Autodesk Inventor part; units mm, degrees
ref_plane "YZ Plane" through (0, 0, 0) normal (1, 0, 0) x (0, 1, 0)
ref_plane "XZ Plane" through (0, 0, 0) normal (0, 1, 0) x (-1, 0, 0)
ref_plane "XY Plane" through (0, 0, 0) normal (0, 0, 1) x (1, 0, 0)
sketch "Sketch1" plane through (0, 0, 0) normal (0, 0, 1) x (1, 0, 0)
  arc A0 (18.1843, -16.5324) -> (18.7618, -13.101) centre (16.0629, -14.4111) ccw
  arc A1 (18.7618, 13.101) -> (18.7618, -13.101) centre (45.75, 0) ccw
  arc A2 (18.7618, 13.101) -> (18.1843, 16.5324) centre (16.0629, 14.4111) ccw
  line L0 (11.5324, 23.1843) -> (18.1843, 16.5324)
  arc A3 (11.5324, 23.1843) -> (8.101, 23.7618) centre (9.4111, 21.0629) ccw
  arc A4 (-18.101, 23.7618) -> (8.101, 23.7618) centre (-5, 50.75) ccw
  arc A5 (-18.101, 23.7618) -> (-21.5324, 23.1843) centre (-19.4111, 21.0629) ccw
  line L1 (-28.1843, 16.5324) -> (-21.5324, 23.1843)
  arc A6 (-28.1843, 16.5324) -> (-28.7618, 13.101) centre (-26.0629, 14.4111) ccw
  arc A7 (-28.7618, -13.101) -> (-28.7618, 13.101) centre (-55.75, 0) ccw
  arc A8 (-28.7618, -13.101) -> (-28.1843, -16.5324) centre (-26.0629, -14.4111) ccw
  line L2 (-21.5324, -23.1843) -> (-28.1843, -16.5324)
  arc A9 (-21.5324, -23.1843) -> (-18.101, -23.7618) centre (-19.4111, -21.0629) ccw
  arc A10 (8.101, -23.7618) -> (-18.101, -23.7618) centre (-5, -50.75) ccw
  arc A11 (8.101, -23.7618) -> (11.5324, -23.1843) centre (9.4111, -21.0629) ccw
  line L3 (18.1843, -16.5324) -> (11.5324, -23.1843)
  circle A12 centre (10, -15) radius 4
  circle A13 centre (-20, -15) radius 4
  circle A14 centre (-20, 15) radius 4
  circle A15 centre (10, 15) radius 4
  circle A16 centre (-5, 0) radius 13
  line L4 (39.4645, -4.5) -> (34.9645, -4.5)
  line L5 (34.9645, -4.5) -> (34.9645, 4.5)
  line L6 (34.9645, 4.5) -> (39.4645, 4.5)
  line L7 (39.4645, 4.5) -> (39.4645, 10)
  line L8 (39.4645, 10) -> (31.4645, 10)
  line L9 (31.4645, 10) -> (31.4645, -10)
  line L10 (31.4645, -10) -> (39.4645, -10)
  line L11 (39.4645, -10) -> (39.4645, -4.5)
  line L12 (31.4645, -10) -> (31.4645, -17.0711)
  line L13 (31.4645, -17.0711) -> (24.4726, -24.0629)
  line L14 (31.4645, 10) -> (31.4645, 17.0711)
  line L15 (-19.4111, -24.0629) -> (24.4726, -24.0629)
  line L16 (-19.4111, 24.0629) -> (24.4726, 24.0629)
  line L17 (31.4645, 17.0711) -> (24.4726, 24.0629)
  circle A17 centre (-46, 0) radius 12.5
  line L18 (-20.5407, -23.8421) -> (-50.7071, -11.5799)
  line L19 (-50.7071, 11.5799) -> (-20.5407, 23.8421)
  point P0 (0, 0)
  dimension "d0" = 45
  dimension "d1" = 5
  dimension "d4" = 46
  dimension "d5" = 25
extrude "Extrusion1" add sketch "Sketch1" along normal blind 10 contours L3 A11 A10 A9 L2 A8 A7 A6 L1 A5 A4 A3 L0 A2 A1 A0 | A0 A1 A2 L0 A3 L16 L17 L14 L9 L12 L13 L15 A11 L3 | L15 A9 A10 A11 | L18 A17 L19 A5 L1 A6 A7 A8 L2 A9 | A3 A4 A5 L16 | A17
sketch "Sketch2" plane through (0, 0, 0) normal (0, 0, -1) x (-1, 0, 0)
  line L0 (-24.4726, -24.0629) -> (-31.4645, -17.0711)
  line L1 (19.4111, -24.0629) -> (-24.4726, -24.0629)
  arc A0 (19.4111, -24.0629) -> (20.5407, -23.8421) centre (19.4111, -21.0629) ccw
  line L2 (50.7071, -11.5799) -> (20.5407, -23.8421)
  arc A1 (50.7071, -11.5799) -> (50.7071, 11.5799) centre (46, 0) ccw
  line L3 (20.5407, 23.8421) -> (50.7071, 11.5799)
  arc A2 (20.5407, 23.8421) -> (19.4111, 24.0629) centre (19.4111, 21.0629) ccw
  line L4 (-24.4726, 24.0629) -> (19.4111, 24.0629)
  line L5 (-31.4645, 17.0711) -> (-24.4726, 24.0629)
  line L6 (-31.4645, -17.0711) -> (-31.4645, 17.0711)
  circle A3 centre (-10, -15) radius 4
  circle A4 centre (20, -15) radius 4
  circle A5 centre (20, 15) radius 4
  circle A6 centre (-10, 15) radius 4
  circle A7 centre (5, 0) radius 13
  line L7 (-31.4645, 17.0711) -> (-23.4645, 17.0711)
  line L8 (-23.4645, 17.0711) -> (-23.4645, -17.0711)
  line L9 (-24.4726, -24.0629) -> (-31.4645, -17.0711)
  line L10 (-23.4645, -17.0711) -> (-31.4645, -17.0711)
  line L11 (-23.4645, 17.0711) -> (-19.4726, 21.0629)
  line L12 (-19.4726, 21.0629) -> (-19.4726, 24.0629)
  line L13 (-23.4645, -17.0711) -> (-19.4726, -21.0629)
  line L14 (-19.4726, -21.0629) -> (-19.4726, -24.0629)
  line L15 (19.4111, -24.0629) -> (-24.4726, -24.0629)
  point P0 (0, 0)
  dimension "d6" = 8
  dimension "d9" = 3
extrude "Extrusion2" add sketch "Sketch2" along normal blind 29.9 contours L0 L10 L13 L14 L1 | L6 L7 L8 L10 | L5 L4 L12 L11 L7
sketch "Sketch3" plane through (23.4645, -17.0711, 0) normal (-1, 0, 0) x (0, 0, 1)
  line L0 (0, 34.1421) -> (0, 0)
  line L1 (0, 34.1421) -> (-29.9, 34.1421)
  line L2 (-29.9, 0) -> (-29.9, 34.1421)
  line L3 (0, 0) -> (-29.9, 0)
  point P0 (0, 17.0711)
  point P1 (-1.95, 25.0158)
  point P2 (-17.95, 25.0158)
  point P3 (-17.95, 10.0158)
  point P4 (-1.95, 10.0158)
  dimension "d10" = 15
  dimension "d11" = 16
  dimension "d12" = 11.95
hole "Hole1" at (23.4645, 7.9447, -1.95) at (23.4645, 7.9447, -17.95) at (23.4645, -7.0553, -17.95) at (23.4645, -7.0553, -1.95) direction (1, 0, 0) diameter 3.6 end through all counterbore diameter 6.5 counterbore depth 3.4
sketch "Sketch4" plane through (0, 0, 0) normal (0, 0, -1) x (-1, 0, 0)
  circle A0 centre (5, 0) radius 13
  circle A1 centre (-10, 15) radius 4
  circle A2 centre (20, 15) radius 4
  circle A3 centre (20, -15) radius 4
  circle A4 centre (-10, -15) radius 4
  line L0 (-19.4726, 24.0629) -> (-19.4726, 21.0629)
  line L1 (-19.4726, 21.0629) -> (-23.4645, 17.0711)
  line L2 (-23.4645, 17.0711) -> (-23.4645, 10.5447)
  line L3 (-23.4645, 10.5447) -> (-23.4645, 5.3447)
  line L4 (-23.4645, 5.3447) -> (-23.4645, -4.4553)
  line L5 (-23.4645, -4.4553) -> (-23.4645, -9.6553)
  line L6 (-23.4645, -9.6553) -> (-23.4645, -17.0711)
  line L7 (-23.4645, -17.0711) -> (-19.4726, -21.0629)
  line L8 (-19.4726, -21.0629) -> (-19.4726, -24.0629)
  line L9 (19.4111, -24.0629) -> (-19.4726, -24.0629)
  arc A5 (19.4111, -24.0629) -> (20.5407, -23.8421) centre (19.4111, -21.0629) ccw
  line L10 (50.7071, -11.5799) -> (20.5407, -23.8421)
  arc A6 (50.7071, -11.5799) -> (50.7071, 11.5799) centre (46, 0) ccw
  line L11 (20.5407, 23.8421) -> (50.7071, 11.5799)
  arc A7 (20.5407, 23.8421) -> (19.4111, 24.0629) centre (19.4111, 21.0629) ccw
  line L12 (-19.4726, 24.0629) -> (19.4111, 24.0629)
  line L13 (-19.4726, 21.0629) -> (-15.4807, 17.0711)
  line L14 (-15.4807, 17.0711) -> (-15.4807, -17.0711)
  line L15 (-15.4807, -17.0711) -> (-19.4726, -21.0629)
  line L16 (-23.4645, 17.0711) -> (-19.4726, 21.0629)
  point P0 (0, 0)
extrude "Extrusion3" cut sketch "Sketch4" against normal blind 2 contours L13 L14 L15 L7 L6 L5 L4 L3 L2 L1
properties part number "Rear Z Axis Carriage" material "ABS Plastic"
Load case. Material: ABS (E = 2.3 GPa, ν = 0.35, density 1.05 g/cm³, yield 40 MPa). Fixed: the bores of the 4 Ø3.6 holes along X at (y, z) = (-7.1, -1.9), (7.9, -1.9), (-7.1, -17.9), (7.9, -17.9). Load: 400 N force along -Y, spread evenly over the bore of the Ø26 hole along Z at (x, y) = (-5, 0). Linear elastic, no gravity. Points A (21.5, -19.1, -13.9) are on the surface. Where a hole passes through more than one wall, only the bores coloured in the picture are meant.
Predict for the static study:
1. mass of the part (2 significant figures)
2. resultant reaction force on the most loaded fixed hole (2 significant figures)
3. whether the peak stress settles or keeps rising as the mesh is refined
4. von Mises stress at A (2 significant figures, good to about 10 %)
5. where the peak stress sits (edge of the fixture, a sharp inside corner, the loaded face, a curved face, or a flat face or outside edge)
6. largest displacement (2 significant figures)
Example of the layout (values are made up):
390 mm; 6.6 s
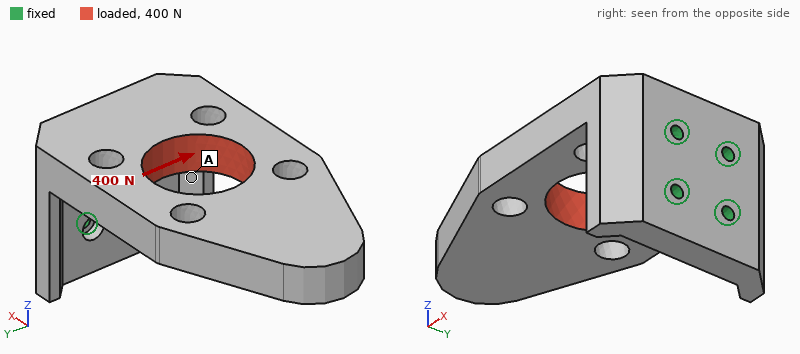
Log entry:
41 g; 680 N; keeps rising; 4.5 MPa; edge of the fixture; 1.2 mm
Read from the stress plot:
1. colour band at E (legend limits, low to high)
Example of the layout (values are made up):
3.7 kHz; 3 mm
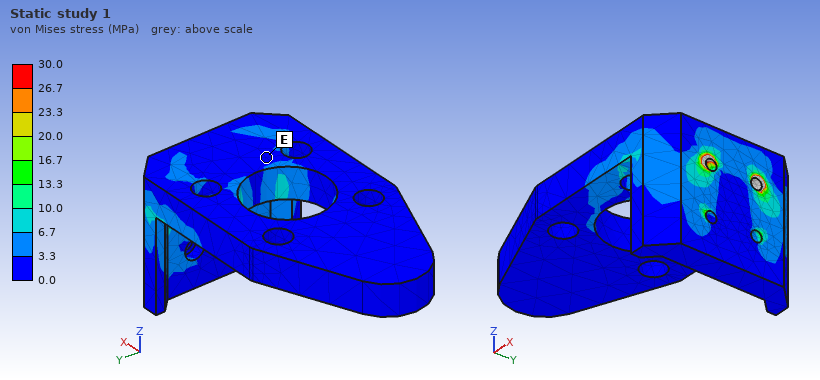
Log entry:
0.0 to 3.3 MPa
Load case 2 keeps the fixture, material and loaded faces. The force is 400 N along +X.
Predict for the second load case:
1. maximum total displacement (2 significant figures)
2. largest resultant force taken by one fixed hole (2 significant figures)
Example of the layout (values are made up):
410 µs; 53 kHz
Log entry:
0.40 mm; 260 N
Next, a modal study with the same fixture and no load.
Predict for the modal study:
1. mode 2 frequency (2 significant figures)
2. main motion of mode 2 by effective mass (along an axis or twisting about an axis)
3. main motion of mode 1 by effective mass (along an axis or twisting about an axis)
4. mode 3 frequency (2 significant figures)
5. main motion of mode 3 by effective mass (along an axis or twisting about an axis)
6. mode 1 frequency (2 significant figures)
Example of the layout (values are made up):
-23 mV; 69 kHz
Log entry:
580 Hz; along Y; along Z; 1200 Hz; twisting about X; 250 Hz
